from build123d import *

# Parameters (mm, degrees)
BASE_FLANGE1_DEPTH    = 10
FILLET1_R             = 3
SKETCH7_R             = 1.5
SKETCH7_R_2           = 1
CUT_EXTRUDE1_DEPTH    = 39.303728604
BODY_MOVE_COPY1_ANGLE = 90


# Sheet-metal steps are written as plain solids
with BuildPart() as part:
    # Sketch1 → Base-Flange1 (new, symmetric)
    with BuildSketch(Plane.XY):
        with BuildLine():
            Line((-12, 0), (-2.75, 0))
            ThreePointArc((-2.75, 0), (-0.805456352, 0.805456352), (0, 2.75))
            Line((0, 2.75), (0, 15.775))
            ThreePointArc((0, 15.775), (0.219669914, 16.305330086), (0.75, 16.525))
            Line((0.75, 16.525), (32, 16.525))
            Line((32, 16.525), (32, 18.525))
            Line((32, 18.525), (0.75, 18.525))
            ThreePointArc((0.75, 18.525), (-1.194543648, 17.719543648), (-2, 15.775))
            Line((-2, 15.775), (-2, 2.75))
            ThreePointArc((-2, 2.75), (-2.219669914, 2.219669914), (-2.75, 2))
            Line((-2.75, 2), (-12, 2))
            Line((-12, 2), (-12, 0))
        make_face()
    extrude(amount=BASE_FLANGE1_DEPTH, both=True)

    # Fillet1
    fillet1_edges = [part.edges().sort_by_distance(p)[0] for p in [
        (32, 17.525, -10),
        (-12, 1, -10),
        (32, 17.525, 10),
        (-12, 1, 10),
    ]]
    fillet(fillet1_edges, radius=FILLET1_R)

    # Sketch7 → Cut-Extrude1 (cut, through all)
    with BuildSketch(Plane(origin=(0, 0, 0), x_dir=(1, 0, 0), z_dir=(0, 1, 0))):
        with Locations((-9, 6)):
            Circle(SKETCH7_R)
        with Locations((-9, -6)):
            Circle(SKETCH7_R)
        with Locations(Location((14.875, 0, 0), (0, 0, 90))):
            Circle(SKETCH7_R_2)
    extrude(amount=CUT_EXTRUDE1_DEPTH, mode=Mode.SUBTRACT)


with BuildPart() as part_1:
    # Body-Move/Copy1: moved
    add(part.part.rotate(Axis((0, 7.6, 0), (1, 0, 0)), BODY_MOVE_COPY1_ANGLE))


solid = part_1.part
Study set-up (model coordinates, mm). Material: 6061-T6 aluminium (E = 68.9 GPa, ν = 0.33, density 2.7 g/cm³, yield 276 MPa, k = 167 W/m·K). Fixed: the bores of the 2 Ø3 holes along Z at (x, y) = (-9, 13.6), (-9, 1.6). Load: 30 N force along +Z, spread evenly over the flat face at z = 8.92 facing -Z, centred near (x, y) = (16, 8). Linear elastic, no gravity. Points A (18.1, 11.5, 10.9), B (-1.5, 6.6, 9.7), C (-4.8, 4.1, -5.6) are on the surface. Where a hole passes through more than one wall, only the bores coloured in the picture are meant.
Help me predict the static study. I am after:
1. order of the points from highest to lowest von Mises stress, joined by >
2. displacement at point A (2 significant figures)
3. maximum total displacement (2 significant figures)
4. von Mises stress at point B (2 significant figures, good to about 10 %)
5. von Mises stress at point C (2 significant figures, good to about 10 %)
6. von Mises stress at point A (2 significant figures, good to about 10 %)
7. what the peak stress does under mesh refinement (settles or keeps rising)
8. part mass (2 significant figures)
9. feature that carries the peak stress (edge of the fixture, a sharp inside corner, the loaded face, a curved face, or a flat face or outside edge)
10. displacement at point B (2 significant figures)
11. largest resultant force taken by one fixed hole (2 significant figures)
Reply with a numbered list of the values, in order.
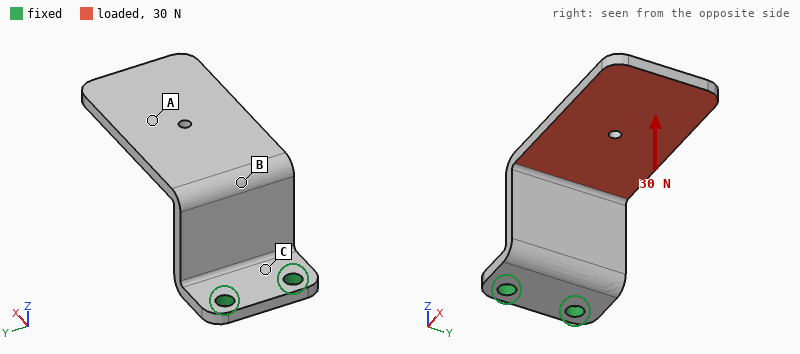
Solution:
1. C > B > A
2. 0.37 mm
3. 0.61 mm
4. 26 MPa
5. 42 MPa
6. 6.9 MPa
7. keeps rising
8. 6.2 g
9. edge of the fixture
10. 0.14 mm
11. 17 N
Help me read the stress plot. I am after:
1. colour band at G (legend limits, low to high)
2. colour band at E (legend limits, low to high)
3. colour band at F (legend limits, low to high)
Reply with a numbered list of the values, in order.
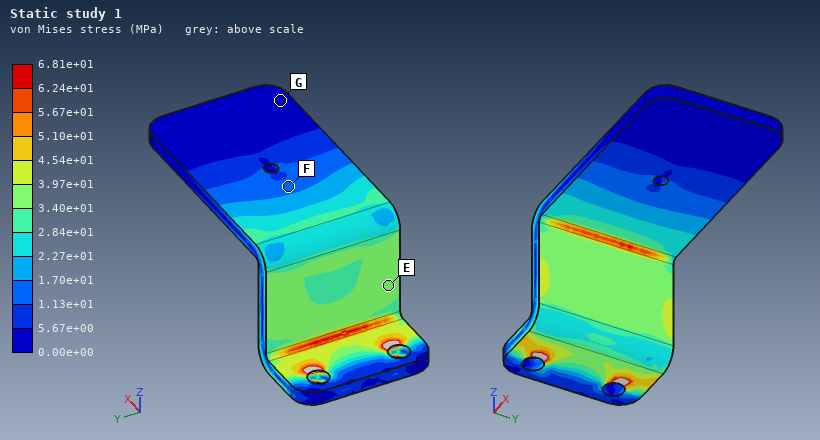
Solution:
1. 0.00e+00 to 5.67e+00 MPa
2. 3.40e+01 to 3.97e+01 MPa
3. 1.13e+01 to 1.70e+01 MPa
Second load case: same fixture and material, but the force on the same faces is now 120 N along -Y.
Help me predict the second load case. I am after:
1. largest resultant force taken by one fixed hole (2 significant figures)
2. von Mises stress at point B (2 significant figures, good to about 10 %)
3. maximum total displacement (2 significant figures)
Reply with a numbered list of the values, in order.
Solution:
1. 260 N
2. 66 MPa
3. 0.58 mm
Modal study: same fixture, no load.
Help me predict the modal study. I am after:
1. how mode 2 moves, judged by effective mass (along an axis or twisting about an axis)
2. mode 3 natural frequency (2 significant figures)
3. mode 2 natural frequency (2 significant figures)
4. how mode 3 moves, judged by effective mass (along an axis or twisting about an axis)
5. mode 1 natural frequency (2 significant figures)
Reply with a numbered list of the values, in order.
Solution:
1. along Y
2. 2400 Hz
3. 1500 Hz
4. along X
5. 700 Hz
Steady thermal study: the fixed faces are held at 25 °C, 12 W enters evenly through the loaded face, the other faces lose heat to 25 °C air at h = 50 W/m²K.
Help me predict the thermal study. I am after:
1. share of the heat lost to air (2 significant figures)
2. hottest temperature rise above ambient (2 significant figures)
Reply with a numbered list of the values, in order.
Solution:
1. 24 %
2. 57 K
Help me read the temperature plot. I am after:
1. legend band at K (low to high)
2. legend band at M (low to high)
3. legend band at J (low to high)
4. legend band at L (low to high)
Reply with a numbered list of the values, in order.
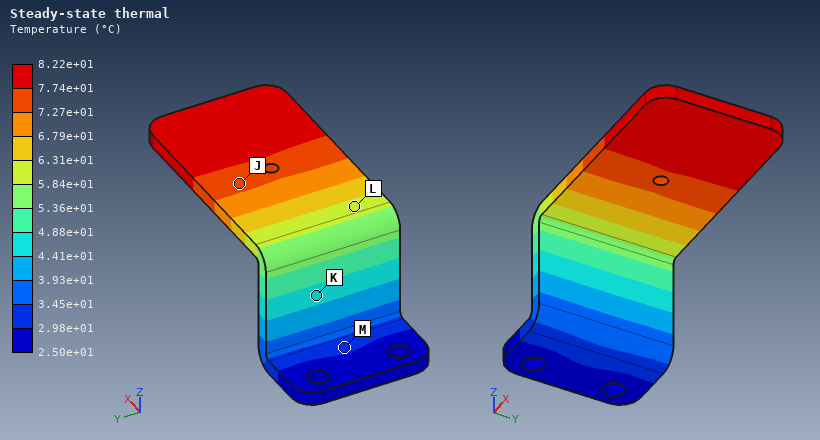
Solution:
1. 4.41e+01 to 4.88e+01 °C
2. 2.98e+01 to 3.45e+01 °C
3. 7.27e+01 to 7.74e+01 °C
4. 5.84e+01 to 6.31e+01 °C
